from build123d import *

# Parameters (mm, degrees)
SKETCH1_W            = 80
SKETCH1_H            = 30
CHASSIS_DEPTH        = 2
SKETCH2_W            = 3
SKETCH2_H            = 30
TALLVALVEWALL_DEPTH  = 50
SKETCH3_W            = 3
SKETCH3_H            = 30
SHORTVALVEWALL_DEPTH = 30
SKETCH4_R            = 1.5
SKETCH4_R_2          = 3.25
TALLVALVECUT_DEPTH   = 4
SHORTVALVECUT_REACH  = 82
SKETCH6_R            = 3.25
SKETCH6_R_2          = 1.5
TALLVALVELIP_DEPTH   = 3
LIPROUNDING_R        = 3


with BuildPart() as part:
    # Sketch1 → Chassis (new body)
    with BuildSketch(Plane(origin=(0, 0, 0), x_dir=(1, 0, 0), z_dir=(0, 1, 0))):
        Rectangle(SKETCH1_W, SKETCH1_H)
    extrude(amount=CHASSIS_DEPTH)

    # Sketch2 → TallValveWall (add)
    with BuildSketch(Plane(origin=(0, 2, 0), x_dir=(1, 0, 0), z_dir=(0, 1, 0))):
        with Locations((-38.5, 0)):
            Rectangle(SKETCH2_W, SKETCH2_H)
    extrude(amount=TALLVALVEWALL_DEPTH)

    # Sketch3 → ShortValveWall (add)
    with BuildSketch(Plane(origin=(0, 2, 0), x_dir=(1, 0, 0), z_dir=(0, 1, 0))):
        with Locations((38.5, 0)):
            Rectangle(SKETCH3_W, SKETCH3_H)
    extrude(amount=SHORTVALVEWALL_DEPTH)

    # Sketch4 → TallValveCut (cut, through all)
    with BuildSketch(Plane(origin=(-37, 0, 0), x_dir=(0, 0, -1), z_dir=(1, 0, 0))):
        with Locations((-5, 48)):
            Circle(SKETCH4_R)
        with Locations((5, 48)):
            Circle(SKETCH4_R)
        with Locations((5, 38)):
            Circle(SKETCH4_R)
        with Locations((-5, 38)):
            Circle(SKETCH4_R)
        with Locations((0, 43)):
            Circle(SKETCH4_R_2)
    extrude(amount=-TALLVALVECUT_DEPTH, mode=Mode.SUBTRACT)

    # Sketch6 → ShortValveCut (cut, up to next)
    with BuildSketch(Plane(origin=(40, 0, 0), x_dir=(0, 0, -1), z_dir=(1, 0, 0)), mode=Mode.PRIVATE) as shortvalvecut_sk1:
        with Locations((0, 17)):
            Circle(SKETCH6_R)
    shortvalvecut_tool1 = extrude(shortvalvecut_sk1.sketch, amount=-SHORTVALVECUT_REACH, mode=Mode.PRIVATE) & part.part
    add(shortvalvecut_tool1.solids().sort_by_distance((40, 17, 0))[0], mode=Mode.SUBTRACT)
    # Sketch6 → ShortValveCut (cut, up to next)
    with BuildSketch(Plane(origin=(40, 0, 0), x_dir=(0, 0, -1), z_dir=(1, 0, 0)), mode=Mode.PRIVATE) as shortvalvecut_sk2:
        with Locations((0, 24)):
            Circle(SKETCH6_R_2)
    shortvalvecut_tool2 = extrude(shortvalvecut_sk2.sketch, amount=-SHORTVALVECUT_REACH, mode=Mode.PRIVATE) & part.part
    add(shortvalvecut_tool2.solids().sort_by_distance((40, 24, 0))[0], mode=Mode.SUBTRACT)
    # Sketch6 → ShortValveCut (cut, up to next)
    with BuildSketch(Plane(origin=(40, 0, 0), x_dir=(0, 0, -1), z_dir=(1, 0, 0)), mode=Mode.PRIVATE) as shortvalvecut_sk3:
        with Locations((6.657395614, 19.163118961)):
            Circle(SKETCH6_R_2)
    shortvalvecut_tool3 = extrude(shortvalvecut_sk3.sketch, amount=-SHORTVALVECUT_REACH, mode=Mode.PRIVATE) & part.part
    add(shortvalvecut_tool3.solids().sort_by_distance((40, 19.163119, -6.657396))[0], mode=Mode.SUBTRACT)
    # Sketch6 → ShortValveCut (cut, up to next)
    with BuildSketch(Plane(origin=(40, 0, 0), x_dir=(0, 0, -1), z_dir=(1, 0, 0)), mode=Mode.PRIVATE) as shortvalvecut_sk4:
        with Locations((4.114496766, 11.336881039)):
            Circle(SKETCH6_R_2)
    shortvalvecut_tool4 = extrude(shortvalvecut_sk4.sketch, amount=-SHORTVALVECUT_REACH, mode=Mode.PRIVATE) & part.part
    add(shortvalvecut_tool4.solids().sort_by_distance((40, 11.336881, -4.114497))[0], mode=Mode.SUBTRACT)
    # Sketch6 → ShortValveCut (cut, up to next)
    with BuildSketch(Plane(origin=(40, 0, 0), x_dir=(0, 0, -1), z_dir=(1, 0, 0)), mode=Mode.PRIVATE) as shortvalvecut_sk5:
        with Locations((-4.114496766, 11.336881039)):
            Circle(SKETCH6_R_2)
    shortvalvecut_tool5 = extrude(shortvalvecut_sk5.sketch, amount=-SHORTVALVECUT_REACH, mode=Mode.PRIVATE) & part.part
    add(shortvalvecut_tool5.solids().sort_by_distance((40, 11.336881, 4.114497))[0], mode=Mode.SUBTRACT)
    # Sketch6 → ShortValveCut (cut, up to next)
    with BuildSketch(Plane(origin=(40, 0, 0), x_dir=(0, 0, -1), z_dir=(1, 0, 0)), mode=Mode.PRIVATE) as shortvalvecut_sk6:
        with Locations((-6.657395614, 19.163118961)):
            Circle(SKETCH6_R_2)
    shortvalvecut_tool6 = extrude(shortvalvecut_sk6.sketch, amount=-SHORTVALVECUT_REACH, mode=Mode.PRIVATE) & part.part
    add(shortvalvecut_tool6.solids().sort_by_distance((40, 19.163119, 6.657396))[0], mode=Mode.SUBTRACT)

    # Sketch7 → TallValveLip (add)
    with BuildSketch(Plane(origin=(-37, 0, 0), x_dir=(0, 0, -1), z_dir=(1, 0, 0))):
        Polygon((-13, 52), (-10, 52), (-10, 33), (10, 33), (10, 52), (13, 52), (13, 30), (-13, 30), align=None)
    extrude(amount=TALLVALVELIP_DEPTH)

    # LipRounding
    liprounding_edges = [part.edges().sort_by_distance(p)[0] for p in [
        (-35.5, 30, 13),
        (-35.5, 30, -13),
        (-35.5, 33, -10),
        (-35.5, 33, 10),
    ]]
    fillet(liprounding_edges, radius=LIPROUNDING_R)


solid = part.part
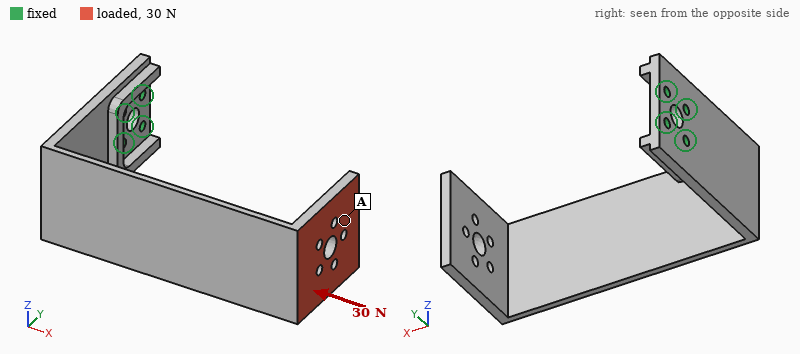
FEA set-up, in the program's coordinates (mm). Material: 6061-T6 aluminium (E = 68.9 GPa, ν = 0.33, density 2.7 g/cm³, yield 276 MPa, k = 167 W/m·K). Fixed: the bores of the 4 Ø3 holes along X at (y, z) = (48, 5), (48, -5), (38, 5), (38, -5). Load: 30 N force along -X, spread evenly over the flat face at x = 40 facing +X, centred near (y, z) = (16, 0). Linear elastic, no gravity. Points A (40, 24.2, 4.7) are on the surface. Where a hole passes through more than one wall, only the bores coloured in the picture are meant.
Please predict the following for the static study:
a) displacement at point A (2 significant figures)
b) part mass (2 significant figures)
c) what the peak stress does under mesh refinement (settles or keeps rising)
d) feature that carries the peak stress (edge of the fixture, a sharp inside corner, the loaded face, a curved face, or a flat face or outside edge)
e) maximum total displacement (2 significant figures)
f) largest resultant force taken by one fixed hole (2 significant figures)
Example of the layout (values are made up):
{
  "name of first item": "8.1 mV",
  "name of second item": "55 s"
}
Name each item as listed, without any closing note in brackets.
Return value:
{
  "displacement at point A": "1.1 mm",
  "part mass": "33 g",
  "what the peak stress does under mesh refinement": "keeps rising",
  "feature that carries the peak stress": "edge of the fixture",
  "maximum total displacement": "1.2 mm",
  "largest resultant force taken by one fixed hole": "32 N"
}
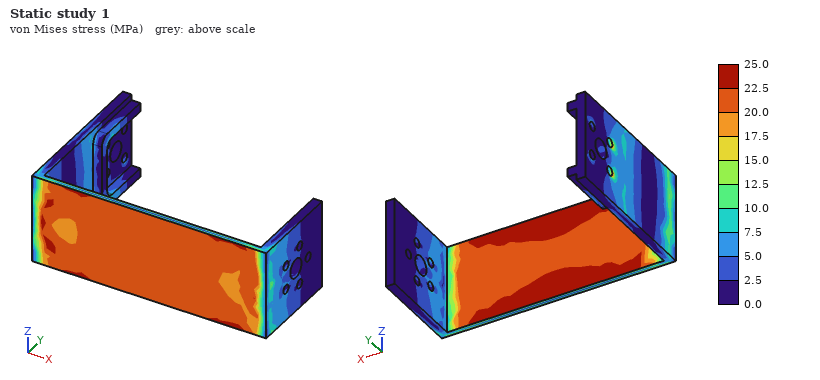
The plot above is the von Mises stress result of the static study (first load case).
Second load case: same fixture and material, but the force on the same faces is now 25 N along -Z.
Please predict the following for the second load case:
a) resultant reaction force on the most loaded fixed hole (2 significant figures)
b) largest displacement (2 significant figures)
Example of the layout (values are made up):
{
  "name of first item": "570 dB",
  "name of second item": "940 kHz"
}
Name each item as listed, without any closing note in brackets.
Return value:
{
  "resultant reaction force on the most loaded fixed hole": "170 N",
  "largest displacement": "1.1 mm"
}
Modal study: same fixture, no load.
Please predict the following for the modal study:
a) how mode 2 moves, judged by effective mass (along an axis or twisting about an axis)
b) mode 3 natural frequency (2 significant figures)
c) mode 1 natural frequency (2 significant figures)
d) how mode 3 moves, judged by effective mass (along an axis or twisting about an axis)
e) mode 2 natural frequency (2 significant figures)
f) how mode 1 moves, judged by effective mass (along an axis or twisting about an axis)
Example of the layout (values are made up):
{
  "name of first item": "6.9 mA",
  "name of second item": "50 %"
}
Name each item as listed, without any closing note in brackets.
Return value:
{
  "how mode 2 moves, judged by effective mass": "along Z",
  "mode 3 natural frequency": "530 Hz",
  "mode 1 natural frequency": "130 Hz",
  "how mode 3 moves, judged by effective mass": "along X",
  "mode 2 natural frequency": "270 Hz",
  "how mode 1 moves, judged by effective mass": "along Y"
}
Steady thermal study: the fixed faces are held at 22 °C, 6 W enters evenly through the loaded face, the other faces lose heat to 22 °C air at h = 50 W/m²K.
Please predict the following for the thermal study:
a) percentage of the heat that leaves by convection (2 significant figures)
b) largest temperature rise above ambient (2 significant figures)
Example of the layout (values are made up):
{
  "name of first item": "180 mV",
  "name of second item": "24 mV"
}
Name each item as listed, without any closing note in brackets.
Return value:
{
  "percentage of the heat that leaves by convection": "78 %",
  "largest temperature rise above ambient": "27 K"
}
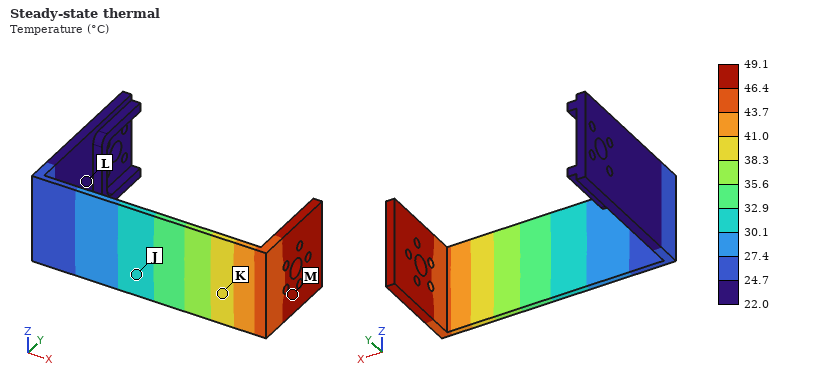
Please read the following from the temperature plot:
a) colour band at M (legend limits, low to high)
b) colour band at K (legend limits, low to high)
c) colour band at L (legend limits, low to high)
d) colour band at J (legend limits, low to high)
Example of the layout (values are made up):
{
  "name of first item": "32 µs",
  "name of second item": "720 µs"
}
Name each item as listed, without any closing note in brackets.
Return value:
{
  "colour band at M": "46.4 to 49.1 °C",
  "colour band at K": "38.3 to 41.0 °C",
  "colour band at L": "22.0 to 24.7 °C",
  "colour band at J": "30.1 to 32.9 °C"
}
